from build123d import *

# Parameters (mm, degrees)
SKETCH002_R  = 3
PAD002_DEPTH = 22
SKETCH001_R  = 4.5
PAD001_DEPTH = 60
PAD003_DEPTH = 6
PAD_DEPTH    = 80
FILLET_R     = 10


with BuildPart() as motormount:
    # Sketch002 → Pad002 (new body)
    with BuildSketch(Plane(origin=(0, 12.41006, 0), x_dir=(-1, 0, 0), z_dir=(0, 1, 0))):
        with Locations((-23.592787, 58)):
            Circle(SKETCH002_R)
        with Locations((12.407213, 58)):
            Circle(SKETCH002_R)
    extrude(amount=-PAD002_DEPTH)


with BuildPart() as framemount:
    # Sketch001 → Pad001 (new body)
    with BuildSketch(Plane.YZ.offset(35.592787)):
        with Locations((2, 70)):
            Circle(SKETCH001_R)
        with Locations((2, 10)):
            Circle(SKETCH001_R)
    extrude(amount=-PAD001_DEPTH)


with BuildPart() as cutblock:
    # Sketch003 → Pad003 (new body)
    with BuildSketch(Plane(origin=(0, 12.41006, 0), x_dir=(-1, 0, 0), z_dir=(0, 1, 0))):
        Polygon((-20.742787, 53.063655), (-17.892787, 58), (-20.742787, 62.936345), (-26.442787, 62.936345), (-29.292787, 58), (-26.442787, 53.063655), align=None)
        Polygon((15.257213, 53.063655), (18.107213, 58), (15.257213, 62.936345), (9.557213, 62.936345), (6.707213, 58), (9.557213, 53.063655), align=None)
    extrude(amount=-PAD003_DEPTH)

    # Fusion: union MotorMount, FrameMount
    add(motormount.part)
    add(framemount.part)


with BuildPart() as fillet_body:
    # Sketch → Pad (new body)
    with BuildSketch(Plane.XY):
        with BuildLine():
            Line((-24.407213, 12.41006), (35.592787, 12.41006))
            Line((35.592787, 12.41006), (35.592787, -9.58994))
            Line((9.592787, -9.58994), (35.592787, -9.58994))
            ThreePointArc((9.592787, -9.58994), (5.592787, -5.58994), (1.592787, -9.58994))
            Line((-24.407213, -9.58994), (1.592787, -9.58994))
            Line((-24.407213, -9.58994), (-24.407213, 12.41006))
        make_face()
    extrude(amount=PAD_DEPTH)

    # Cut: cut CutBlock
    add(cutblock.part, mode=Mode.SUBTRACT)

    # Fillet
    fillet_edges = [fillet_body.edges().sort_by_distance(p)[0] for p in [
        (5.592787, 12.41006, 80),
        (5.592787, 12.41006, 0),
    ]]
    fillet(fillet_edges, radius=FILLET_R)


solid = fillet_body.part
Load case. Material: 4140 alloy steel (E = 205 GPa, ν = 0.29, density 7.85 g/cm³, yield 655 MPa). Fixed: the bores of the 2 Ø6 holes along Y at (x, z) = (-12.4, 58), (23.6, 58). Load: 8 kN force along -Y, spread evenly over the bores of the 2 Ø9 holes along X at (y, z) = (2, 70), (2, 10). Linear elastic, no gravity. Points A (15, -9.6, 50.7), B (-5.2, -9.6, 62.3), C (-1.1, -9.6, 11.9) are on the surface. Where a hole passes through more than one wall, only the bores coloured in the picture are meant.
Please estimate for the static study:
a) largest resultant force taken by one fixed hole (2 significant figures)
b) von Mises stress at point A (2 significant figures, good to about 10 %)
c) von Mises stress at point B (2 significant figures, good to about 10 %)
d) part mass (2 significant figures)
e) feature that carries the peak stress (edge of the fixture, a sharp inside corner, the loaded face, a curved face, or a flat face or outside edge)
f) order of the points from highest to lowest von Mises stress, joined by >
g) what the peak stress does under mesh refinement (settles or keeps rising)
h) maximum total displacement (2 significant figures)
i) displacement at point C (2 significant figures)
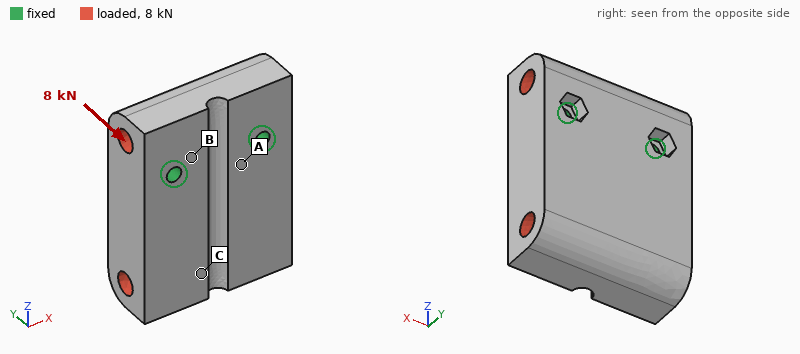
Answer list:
4.0 kN
33 MPa
21 MPa
720 g
edge of the fixture
A > B > C
keeps rising
33 µm
26 µm
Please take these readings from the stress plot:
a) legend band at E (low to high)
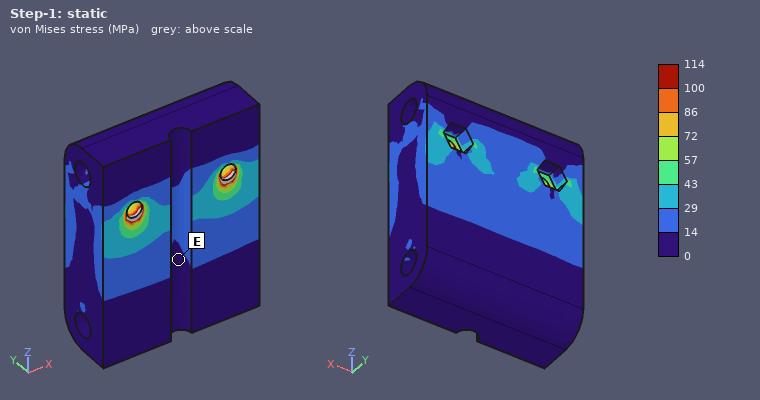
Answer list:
0 to 14 MPa
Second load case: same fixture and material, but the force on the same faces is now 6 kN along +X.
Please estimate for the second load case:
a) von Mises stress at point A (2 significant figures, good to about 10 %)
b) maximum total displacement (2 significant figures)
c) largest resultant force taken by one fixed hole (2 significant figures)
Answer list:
6.8 MPa
5.0 µm
4.1 kN
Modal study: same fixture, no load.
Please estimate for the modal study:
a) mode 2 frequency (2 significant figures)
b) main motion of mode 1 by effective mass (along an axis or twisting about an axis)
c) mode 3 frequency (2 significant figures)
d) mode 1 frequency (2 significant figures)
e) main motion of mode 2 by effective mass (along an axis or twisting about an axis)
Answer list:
8200 Hz
along Y
9300 Hz
3900 Hz
along X
